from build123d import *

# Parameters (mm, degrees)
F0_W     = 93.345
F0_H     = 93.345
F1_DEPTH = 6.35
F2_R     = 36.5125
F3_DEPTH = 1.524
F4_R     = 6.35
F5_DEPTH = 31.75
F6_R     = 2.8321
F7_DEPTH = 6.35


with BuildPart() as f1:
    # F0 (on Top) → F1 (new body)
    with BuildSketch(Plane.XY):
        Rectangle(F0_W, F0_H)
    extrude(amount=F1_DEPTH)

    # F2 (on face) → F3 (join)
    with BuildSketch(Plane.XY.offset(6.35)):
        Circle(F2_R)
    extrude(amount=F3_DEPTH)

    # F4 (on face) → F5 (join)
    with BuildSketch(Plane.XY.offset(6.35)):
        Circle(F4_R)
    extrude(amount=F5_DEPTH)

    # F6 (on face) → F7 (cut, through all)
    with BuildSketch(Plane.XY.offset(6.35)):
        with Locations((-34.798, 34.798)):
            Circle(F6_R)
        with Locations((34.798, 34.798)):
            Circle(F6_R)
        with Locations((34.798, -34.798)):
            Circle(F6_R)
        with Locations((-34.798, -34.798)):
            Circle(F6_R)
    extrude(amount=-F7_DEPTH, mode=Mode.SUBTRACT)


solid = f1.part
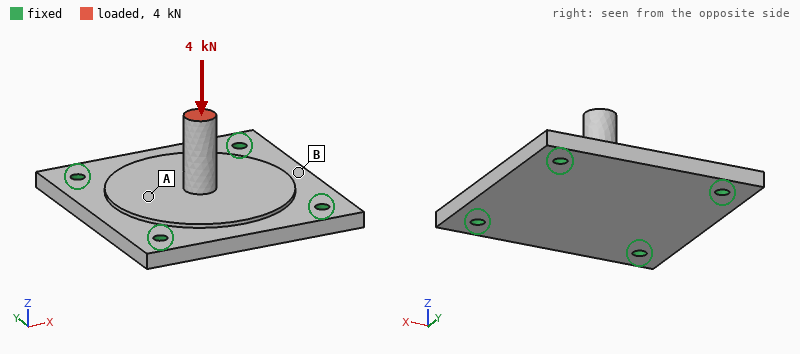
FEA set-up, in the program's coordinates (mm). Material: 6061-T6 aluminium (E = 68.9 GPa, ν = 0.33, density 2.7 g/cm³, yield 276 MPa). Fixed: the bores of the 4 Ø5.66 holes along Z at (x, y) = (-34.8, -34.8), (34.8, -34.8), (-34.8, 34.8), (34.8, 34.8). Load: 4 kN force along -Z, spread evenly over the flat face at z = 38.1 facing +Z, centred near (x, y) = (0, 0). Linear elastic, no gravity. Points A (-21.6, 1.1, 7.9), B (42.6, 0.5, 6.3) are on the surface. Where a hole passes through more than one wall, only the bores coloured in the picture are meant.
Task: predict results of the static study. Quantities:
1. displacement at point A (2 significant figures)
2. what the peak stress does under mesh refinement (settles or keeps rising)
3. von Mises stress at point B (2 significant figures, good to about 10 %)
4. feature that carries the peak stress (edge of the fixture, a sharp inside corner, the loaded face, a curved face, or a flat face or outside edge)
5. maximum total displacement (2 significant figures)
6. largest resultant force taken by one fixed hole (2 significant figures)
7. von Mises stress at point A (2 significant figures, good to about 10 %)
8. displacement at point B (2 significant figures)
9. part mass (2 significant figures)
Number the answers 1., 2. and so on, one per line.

1. 0.066 mm
2. keeps rising
3. 16 MPa
4. edge of the fixture
5. 0.11 mm
6. 1.2 kN
7. 36 MPa
8. 0.022 mm
9. 180 g
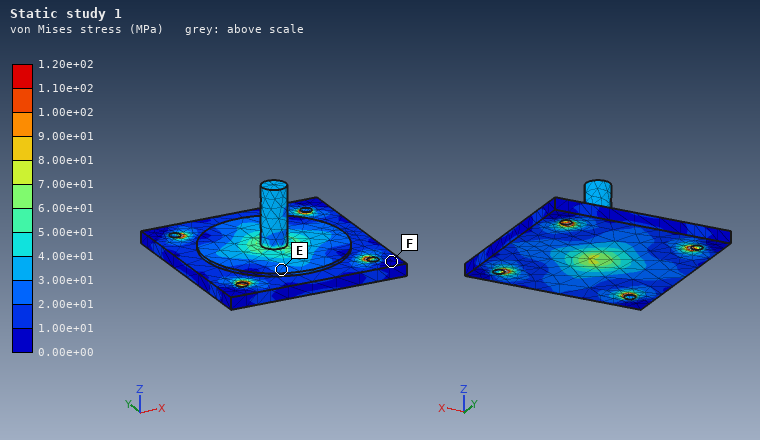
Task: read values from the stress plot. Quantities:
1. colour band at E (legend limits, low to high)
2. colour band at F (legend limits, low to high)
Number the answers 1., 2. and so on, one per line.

1. 2.00e+01 to 3.00e+01 MPa
2. 0.00e+00 to 1.00e+01 MPa
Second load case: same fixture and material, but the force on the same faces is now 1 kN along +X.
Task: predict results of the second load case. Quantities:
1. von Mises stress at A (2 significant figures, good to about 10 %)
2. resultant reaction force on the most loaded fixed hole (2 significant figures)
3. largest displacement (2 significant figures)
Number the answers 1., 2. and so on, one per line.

1. 13 MPa
2. 420 N
3. 0.20 mm
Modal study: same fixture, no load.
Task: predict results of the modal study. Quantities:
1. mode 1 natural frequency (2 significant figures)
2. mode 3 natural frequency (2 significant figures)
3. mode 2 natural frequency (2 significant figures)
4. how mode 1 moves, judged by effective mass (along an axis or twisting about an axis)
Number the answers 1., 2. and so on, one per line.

1. 4400 Hz
2. 6000 Hz
3. 6000 Hz
4. along Z
